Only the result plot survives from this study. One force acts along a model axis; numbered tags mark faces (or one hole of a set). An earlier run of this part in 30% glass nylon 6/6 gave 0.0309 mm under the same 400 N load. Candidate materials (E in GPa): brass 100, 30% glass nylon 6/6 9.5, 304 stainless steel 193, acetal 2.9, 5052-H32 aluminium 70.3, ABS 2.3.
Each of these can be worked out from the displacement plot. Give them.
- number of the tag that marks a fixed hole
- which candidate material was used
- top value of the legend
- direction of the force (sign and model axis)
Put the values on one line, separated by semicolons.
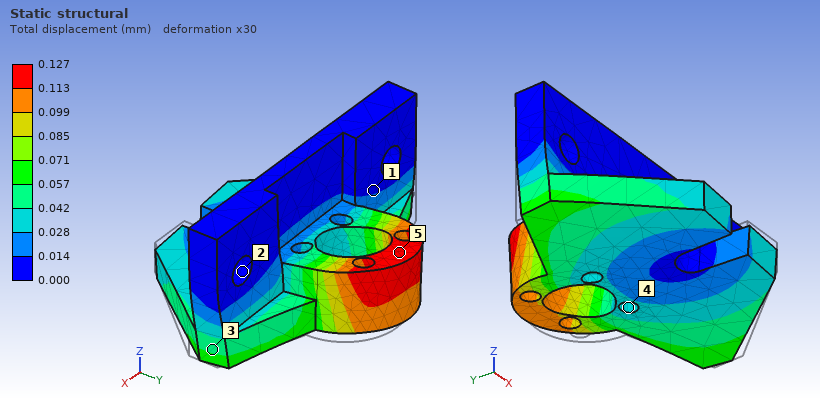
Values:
2; ABS; 0.127 mm; -X
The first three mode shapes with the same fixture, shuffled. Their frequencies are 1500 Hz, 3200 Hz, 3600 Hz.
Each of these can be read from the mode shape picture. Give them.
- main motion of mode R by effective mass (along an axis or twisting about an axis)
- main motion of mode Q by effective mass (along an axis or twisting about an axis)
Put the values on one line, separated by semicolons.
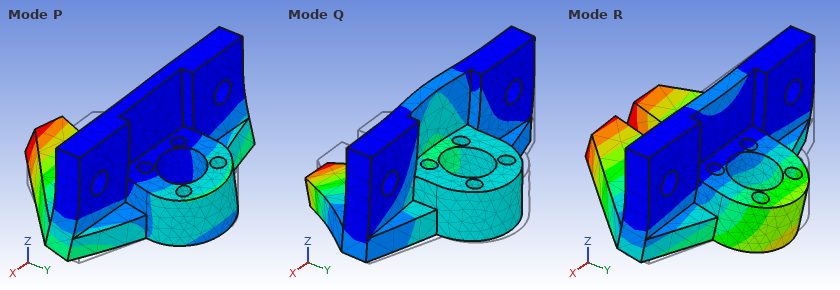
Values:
along Y; along Y
